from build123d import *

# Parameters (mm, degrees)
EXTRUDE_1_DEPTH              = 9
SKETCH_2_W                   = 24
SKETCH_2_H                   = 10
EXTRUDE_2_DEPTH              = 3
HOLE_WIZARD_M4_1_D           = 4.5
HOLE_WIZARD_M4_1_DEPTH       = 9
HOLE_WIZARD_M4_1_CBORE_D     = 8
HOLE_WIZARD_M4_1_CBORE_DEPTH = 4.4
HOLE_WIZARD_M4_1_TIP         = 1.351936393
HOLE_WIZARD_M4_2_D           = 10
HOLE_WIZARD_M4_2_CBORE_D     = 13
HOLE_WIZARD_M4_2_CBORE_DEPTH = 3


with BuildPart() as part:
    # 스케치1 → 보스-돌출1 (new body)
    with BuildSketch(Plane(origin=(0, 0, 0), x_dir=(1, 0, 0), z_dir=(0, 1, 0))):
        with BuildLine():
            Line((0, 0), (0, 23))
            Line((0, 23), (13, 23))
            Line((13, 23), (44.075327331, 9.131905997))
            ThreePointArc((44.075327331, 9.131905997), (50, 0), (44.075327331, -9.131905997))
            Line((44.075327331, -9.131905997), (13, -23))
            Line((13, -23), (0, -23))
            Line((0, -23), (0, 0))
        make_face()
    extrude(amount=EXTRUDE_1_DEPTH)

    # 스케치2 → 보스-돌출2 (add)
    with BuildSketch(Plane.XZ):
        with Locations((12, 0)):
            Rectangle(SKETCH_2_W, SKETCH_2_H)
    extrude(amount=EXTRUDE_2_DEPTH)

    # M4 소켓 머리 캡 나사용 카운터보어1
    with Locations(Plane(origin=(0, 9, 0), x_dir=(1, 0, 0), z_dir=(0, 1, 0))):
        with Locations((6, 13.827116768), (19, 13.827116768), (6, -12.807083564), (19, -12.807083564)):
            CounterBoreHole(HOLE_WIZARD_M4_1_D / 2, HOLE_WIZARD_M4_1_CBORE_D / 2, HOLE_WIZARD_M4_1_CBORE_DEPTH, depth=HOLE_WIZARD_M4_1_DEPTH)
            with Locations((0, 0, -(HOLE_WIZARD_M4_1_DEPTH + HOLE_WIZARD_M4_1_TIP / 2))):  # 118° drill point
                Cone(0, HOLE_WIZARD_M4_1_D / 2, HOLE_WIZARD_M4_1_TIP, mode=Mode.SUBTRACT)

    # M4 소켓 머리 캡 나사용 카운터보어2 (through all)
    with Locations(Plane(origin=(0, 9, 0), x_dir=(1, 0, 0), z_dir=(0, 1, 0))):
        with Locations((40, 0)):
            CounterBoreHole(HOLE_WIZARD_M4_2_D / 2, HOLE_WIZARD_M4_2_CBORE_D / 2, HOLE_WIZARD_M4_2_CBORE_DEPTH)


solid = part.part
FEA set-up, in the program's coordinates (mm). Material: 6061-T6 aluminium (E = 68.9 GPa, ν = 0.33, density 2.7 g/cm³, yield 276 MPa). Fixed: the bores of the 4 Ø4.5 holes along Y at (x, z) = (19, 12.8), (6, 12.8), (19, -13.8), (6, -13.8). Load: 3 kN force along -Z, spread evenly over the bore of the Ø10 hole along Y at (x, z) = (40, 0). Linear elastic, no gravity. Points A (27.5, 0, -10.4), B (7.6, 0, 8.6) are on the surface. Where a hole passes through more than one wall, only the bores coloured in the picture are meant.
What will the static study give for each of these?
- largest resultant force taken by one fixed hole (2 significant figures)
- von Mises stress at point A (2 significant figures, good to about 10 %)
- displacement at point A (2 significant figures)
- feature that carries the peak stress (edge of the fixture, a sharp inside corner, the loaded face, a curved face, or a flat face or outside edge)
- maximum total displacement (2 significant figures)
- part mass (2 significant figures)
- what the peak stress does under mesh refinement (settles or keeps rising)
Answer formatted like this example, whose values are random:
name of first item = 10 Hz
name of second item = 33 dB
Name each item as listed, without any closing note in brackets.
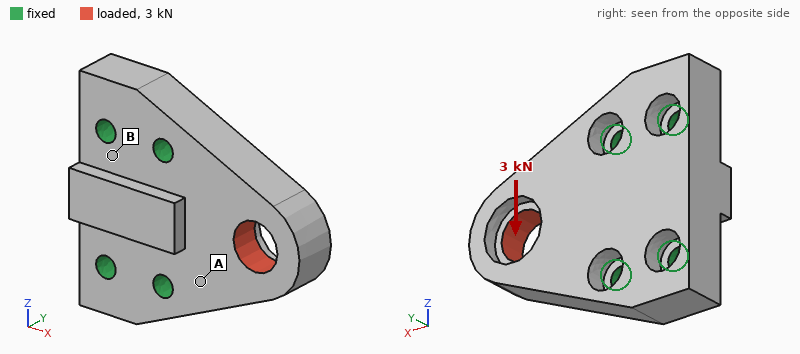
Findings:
largest resultant force taken by one fixed hole = 2.3 kN
von Mises stress at point A = 32 MPa
displacement at point A = 6.0 µm
feature that carries the peak stress = edge of the fixture
maximum total displacement = 33 µm
part mass = 37 g
what the peak stress does under mesh refinement = keeps rising
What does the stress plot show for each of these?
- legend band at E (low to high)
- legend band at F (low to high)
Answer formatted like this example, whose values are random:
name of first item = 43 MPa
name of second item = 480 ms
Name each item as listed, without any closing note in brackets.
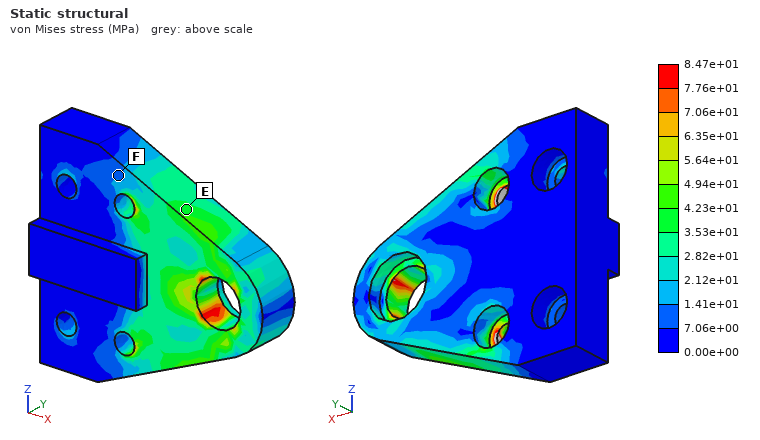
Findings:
legend band at E = 3.53e+01 to 4.23e+01 MPa
legend band at F = 7.06e+00 to 1.41e+01 MPa
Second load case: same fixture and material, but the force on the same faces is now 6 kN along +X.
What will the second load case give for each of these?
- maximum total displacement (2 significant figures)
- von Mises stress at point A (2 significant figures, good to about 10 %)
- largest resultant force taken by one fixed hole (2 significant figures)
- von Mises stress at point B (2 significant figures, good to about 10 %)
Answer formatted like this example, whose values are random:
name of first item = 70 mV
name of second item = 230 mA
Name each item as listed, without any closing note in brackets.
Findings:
maximum total displacement = 36 µm
von Mises stress at point A = 47 MPa
largest resultant force taken by one fixed hole = 2.4 kN
von Mises stress at point B = 15 MPa
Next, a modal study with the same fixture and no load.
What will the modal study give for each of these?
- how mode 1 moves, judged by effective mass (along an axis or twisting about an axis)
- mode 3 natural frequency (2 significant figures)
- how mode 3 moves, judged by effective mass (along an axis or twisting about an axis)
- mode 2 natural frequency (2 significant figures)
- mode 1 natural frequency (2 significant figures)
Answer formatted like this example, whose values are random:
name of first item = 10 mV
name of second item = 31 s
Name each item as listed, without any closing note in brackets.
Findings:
how mode 1 moves, judged by effective mass = along Y
mode 3 natural frequency = 23 kHz
how mode 3 moves, judged by effective mass = along Z
mode 2 natural frequency = 22 kHz
mode 1 natural frequency = 8600 Hz
